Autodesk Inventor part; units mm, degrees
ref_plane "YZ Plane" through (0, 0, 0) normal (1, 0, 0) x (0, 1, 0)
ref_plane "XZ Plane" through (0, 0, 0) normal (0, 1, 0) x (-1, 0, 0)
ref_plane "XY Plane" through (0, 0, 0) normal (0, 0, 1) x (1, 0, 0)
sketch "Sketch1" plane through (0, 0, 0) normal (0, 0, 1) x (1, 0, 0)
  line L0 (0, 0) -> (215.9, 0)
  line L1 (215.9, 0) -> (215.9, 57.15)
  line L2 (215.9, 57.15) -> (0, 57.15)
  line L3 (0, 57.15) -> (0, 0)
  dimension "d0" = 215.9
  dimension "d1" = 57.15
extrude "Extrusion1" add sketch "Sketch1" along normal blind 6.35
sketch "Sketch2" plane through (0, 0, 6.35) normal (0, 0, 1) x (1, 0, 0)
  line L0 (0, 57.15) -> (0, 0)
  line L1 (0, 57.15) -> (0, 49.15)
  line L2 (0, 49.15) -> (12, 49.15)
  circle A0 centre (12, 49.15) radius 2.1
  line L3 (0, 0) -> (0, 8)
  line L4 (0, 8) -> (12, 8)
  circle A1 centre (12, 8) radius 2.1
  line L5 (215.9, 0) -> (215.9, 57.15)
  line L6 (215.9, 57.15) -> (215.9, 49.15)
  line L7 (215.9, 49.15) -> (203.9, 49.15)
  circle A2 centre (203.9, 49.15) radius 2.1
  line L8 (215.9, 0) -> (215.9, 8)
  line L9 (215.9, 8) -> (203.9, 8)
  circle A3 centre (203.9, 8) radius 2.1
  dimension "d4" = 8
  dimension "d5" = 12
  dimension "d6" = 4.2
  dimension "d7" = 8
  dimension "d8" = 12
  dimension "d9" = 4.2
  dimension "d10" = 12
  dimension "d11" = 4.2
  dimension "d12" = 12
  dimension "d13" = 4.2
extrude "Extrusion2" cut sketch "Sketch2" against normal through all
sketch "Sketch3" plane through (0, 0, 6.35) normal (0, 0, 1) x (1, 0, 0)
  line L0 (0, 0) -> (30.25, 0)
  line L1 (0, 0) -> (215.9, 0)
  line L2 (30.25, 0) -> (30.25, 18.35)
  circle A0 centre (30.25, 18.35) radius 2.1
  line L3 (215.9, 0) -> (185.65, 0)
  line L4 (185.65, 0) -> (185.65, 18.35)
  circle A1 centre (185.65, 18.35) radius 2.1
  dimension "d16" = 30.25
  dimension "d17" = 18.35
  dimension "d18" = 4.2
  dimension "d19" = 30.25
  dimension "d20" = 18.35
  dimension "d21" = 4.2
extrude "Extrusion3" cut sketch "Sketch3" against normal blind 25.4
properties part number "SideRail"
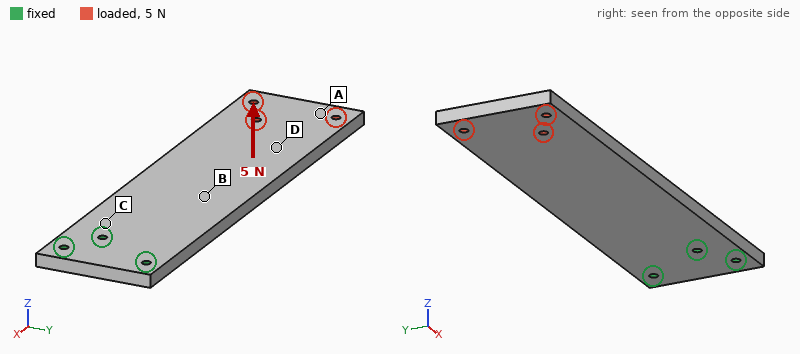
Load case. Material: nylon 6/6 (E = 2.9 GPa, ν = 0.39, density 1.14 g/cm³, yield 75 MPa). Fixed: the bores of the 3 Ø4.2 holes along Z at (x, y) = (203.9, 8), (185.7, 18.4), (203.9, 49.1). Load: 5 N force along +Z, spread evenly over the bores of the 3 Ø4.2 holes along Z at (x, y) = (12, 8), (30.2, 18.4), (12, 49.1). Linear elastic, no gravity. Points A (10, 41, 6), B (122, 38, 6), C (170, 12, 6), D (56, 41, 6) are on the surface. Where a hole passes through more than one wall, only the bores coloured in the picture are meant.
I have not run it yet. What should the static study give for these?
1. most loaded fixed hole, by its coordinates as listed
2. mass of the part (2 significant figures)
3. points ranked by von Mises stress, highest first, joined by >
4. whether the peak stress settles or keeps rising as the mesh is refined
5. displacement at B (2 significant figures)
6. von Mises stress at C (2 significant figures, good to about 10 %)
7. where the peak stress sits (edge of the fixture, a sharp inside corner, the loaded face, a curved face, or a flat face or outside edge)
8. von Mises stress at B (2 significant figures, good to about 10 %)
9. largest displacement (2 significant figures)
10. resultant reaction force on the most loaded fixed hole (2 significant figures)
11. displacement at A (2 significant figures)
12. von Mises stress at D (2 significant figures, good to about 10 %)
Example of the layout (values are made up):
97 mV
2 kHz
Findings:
(185.7, 18.4)
89 g
C > B > D > A
keeps rising
0.47 mm
2.0 MPa
edge of the fixture
1.3 MPa
2.7 mm
30 N
2.5 mm
0.50 MPa
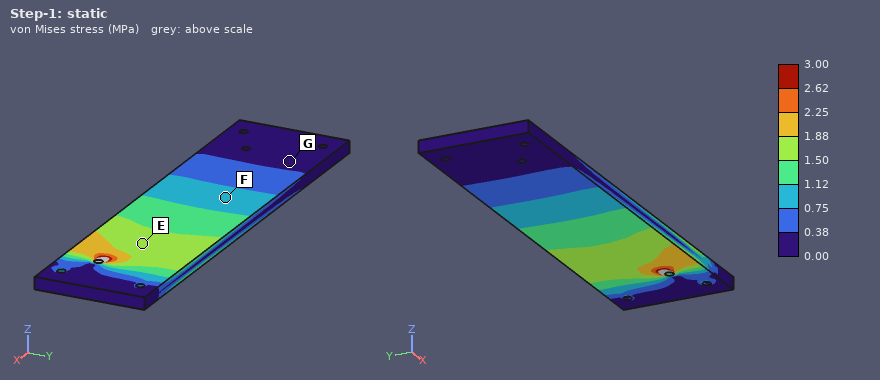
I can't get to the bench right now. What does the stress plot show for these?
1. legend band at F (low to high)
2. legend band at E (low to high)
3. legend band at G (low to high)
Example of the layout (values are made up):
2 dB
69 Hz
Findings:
0.75 to 1.12 MPa
1.50 to 1.88 MPa
0.00 to 0.38 MPa
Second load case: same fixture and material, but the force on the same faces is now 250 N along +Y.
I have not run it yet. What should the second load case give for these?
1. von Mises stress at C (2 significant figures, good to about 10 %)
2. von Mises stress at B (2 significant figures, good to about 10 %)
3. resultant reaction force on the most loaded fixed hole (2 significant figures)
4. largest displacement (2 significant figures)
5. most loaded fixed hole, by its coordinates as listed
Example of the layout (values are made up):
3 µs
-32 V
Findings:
6.4 MPa
2.9 MPa
1.0 kN
2.2 mm
(203.9, 49.1)
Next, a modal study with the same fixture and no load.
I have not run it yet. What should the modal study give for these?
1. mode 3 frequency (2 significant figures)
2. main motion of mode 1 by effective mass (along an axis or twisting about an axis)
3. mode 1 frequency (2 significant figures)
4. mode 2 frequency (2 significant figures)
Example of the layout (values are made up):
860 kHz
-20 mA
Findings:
300 Hz
along Z
47 Hz
270 Hz
